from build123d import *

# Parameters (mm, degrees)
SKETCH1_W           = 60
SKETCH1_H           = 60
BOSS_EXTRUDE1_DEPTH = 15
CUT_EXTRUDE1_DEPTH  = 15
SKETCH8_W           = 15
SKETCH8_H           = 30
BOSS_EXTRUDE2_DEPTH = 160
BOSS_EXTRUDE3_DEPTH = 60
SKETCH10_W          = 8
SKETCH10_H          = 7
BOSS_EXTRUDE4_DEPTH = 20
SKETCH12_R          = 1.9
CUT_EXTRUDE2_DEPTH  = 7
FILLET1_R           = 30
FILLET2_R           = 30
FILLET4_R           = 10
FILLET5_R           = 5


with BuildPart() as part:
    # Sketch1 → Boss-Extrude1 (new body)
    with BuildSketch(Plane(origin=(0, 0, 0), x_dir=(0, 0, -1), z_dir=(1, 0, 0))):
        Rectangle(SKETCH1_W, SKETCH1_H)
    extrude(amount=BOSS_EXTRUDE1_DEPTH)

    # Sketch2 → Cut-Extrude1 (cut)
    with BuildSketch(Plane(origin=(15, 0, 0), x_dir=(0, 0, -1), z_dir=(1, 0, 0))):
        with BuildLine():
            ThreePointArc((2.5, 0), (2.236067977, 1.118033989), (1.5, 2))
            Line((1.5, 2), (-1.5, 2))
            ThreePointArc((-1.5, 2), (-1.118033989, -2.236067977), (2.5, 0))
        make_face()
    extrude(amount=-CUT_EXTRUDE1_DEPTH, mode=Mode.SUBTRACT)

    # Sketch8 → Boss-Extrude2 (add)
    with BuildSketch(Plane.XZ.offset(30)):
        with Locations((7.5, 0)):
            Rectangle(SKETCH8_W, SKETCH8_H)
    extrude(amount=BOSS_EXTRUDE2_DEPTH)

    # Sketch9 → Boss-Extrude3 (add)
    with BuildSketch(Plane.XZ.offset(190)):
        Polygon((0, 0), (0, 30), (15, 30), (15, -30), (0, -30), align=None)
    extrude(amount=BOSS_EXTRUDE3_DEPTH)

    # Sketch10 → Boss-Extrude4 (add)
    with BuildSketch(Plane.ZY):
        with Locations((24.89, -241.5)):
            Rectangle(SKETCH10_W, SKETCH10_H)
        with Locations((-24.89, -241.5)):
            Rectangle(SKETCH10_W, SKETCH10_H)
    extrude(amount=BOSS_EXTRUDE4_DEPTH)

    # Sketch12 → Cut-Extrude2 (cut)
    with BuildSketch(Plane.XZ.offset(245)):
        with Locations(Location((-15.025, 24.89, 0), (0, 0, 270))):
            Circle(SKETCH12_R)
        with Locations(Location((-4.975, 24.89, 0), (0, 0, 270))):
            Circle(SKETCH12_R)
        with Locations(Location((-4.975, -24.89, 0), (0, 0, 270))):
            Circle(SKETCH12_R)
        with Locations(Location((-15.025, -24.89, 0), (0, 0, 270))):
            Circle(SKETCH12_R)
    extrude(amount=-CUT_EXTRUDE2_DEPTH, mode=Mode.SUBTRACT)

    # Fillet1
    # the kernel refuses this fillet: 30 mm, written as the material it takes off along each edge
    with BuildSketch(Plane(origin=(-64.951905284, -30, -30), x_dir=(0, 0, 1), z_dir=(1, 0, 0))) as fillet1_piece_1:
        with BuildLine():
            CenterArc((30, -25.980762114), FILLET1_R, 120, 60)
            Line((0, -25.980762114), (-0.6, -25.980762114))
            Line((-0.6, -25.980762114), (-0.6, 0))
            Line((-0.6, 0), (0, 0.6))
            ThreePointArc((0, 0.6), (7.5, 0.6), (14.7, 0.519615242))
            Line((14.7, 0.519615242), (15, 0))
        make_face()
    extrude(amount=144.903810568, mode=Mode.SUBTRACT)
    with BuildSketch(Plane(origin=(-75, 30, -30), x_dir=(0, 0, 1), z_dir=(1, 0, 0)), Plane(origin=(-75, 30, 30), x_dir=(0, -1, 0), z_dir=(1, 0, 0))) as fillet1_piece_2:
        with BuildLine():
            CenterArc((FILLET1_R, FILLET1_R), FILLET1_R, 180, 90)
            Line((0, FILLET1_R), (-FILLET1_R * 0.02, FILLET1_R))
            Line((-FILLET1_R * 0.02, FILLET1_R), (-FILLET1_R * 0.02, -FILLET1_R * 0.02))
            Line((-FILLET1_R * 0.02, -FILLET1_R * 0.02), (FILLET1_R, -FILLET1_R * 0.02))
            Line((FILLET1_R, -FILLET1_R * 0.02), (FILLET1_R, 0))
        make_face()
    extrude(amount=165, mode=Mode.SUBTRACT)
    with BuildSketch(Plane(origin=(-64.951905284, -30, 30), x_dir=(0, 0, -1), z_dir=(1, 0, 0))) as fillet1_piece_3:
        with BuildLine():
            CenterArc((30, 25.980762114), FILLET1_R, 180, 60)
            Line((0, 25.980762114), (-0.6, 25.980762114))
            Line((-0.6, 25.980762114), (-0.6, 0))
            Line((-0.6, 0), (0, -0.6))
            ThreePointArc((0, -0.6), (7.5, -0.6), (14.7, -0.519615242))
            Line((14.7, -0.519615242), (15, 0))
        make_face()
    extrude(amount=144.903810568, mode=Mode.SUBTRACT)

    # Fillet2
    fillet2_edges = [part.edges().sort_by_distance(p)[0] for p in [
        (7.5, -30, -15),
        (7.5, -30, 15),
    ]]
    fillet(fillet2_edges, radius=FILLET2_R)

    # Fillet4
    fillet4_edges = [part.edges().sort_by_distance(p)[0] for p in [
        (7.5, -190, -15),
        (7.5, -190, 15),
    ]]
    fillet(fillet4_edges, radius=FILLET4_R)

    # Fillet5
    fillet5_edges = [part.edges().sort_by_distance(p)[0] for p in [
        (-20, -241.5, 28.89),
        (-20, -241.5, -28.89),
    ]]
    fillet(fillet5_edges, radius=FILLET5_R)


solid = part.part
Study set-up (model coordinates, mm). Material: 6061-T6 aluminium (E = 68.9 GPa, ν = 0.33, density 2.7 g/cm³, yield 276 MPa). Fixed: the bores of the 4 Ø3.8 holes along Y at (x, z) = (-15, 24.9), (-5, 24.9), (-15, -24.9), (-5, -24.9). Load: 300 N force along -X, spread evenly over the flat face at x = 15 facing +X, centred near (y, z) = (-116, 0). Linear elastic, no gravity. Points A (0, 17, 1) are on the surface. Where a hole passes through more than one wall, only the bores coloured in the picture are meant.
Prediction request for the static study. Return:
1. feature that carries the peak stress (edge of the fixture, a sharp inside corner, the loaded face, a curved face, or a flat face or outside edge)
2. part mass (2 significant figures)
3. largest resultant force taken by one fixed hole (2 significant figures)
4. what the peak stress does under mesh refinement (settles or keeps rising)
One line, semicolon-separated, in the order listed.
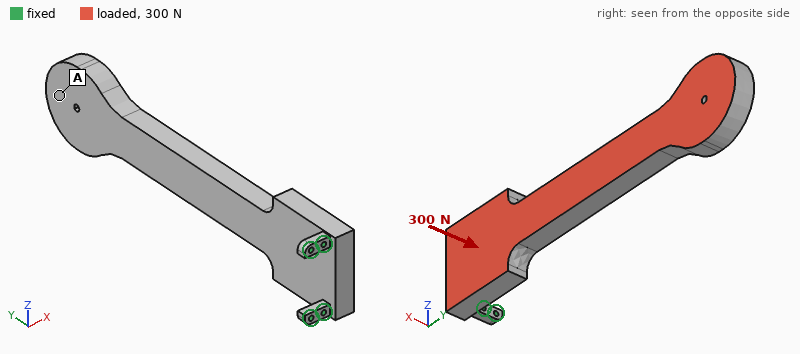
edge of the fixture; 470 g; 200 N; keeps rising
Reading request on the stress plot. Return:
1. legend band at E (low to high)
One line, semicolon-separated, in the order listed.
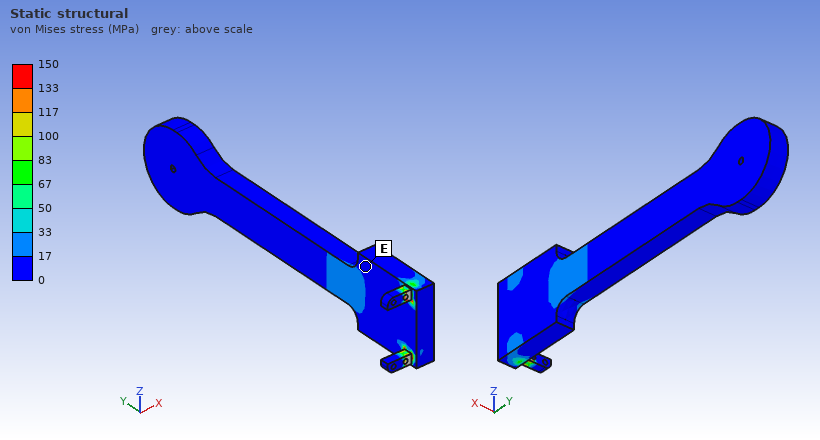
0 to 17 MPa
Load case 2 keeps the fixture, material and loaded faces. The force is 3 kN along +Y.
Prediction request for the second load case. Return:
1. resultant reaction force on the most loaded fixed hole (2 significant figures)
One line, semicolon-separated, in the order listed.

1.7 kN
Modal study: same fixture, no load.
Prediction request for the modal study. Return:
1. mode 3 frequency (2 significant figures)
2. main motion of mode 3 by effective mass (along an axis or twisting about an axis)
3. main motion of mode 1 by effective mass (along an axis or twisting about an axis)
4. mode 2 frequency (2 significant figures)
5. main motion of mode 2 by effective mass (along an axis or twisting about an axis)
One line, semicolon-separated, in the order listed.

740 Hz; along X; along X; 330 Hz; along Z
